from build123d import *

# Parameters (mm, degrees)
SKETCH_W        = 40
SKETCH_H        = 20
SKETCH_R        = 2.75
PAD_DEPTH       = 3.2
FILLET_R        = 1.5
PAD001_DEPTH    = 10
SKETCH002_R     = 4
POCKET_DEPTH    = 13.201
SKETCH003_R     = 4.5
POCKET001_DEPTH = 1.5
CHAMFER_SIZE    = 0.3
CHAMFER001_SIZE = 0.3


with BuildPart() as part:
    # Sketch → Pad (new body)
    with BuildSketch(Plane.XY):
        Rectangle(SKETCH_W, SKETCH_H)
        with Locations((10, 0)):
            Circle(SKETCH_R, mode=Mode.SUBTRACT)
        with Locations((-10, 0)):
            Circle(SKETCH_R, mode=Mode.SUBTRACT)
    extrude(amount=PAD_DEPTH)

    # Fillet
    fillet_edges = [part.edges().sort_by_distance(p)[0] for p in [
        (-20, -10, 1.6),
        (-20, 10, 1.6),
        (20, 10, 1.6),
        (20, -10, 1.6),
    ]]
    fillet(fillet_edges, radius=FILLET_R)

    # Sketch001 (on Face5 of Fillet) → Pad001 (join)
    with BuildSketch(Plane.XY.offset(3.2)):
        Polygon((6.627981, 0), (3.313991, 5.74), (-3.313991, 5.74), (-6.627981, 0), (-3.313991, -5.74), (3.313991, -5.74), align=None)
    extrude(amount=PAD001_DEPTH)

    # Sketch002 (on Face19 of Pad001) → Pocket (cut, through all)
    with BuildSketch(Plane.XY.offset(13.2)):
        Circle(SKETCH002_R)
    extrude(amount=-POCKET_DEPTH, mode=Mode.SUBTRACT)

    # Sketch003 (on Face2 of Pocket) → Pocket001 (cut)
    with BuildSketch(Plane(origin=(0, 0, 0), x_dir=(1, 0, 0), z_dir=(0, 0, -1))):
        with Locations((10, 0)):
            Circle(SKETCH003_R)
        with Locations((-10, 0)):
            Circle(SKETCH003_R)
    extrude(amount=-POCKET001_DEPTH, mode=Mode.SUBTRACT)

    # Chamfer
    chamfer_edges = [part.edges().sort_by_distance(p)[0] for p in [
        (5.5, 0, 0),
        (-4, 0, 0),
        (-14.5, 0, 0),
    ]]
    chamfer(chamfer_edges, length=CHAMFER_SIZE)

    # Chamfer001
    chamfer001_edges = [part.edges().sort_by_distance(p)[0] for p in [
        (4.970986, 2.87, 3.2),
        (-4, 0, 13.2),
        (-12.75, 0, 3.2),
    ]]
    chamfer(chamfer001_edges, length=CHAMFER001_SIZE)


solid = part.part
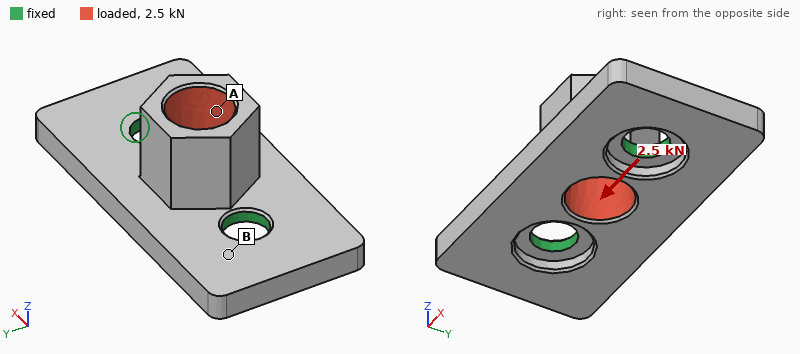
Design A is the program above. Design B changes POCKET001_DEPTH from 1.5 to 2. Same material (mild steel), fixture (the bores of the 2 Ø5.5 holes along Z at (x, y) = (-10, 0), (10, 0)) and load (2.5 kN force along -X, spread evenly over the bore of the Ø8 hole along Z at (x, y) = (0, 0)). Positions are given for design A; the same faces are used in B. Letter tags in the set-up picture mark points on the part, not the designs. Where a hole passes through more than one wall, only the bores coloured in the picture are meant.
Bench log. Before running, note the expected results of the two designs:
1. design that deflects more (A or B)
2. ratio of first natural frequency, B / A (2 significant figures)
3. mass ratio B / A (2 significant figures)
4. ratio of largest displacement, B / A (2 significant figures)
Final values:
B
0.78
0.99
1.2
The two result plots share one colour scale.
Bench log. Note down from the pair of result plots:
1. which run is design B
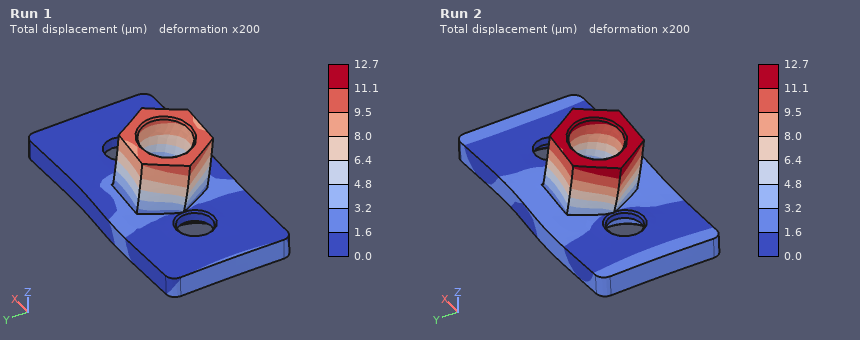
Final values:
Run 2
